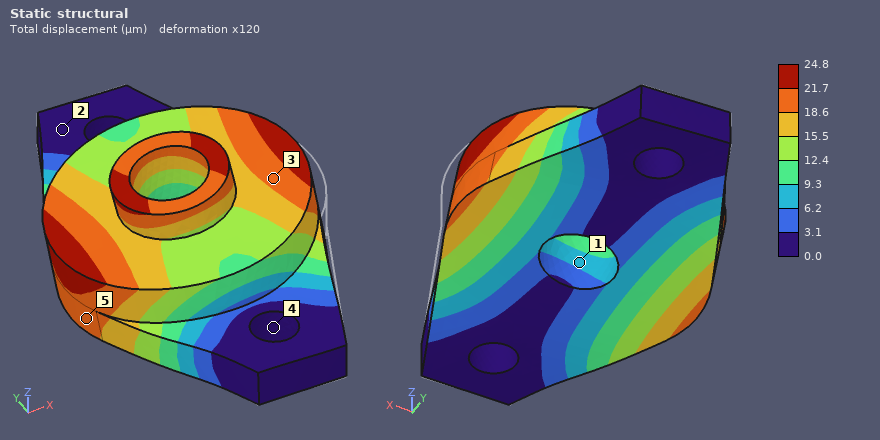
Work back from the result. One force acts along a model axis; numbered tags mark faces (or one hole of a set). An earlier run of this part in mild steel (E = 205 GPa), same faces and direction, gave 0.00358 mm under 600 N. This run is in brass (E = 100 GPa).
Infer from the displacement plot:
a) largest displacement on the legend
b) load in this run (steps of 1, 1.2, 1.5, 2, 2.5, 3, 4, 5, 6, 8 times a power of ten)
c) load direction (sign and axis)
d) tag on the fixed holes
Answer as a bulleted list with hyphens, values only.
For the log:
- 24.8 µm
- 2 kN
- -X
- 4
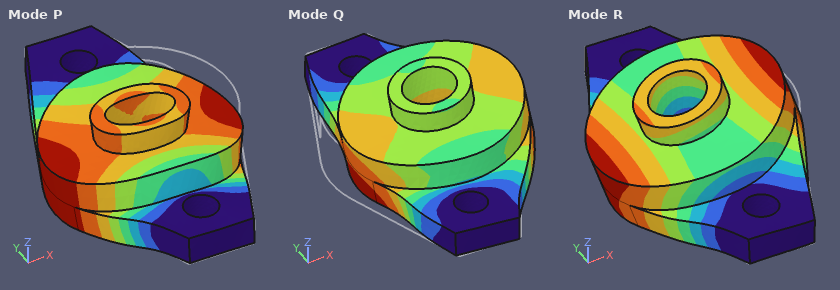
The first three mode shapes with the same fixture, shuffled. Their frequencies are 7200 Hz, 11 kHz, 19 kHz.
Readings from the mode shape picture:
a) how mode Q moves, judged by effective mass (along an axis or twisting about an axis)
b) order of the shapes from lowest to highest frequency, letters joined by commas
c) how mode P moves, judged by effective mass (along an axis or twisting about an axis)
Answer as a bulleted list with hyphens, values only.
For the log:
- along X
- R, P, Q
- along Z
